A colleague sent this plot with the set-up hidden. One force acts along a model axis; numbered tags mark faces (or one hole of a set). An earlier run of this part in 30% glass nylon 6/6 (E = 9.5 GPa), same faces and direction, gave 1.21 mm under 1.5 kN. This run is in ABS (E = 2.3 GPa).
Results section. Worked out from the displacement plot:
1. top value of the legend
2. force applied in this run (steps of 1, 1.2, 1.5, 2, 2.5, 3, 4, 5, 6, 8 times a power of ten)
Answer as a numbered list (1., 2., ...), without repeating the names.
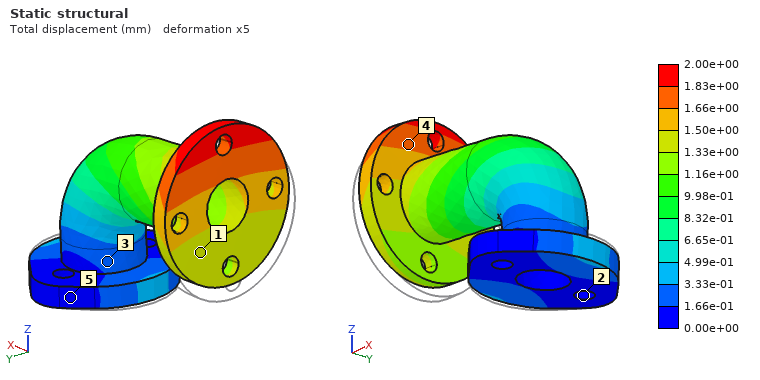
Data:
1. 2.00e+00 mm
2. 600 N
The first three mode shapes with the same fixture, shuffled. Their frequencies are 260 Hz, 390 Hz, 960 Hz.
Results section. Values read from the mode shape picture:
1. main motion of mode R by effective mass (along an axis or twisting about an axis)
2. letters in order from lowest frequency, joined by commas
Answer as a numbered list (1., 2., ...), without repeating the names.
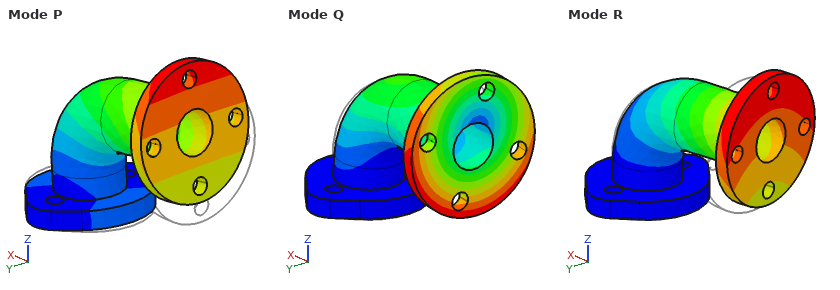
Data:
1. along Y
2. P, R, Q
